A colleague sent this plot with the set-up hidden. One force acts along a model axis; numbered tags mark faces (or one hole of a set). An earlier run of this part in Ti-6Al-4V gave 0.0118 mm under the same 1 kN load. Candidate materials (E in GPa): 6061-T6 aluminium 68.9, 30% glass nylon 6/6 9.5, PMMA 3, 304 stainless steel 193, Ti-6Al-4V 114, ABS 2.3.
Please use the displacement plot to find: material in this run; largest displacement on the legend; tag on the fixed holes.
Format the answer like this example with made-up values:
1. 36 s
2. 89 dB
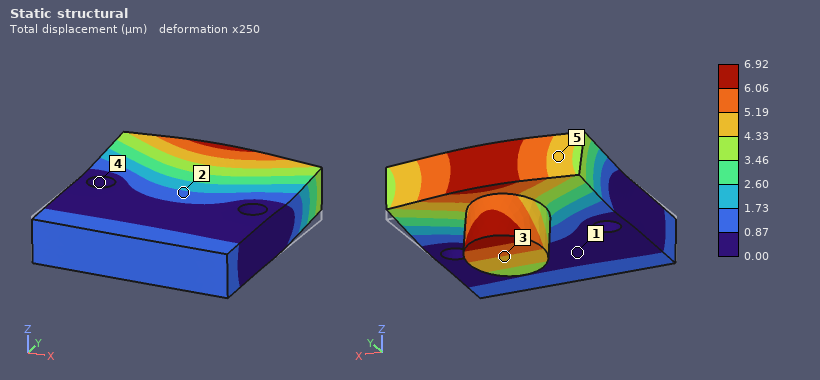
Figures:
1. 304 stainless steel
2. 6.92 µm
3. 4
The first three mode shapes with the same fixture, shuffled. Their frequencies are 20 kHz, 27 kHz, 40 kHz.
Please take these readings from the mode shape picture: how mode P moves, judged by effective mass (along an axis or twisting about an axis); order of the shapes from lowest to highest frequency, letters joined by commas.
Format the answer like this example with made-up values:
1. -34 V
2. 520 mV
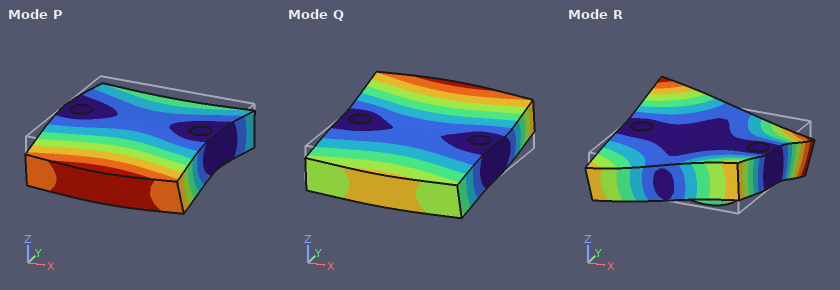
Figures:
1. along Z
2. Q, P, R
